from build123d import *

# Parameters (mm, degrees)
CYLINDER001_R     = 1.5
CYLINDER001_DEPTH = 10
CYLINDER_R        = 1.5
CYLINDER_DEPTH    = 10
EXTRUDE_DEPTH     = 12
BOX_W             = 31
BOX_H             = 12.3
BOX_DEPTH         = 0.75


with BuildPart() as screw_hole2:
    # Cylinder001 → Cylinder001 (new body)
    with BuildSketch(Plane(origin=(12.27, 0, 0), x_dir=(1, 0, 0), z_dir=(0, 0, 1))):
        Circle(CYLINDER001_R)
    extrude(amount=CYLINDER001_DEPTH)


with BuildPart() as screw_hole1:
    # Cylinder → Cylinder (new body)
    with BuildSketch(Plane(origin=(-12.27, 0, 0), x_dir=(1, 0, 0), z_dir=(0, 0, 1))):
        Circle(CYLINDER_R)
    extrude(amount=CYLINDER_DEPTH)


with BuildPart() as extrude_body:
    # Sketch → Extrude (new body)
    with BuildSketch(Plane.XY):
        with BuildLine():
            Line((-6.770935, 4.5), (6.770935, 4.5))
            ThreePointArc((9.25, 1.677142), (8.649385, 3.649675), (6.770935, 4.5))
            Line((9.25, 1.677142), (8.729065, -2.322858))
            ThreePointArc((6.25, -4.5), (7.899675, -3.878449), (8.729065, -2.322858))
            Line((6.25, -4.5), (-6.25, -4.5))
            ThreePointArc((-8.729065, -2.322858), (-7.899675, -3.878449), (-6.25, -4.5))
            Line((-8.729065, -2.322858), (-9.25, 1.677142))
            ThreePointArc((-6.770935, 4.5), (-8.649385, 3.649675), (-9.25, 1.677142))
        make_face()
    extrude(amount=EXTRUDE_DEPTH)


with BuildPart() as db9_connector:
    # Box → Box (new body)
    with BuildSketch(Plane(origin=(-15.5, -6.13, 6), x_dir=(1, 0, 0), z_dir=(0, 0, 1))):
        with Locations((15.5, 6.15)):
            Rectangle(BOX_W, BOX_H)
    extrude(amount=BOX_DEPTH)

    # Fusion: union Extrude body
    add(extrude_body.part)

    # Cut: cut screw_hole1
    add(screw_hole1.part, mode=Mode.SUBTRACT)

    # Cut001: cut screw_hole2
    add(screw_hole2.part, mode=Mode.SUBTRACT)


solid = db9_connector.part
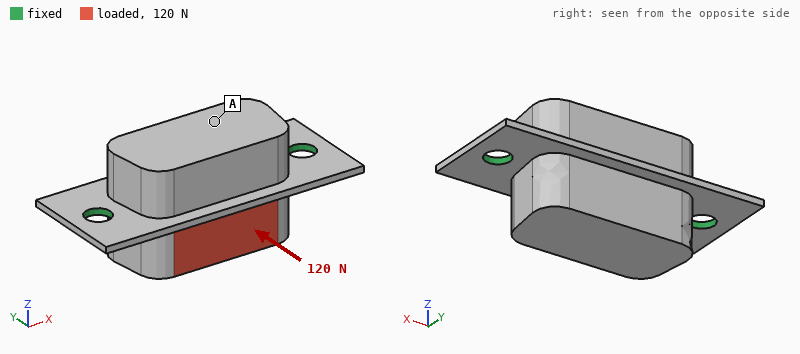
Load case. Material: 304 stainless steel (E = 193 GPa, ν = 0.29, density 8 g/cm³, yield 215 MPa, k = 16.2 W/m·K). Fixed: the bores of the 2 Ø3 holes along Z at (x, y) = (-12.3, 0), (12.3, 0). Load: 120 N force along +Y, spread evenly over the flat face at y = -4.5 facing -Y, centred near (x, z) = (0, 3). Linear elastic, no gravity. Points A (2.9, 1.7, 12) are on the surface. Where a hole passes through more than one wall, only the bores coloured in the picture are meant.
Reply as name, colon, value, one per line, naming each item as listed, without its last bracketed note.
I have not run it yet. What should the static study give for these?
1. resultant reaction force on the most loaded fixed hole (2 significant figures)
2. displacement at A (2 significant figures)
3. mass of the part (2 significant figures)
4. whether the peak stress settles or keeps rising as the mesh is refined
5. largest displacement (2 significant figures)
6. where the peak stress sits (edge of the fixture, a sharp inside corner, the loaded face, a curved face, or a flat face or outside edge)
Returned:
resultant reaction force on the most loaded fixed hole: 60 N
displacement at A: 11 µm
mass of the part: 16 g
whether the peak stress settles or keeps rising as the mesh is refined: keeps rising
largest displacement: 17 µm
where the peak stress sits: edge of the fixture
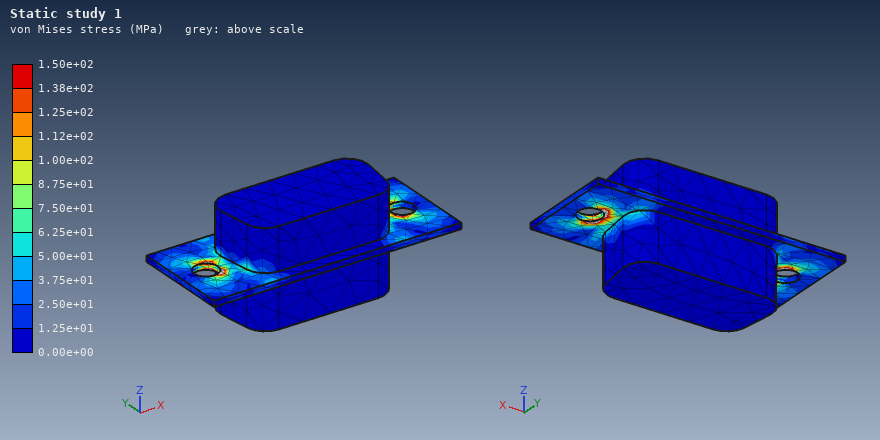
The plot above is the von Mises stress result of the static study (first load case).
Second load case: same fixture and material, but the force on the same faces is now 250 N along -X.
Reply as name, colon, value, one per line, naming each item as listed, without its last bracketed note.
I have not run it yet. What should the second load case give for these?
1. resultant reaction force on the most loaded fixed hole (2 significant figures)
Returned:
resultant reaction force on the most loaded fixed hole: 140 N
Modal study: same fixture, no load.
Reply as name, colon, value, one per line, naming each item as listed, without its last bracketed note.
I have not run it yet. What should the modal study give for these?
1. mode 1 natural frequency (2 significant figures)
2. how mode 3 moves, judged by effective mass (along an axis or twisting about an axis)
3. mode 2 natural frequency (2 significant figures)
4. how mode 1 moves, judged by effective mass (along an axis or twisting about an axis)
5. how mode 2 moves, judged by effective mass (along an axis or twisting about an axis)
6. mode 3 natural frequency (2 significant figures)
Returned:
mode 1 natural frequency: 4100 Hz
how mode 3 moves, judged by effective mass: twisting about Y
mode 2 natural frequency: 10 kHz
how mode 1 moves, judged by effective mass: twisting about X
how mode 2 moves, judged by effective mass: along Z
mode 3 natural frequency: 17 kHz
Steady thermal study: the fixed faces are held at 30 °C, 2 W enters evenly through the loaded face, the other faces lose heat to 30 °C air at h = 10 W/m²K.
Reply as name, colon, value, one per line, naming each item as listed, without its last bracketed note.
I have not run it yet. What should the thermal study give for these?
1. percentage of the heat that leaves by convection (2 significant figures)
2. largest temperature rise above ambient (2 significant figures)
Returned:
percentage of the heat that leaves by convection: 14 %
largest temperature rise above ambient: 34 K
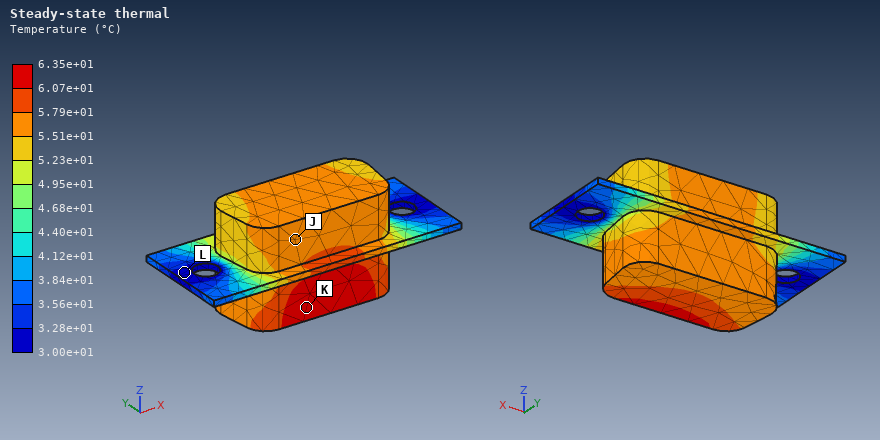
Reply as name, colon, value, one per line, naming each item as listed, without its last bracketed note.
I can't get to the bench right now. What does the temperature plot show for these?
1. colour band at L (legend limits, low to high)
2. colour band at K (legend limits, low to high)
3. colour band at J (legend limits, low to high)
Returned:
colour band at L: 3.00e+01 to 3.28e+01 °C
colour band at K: 6.07e+01 to 6.35e+01 °C
colour band at J: 5.51e+01 to 5.79e+01 °C
